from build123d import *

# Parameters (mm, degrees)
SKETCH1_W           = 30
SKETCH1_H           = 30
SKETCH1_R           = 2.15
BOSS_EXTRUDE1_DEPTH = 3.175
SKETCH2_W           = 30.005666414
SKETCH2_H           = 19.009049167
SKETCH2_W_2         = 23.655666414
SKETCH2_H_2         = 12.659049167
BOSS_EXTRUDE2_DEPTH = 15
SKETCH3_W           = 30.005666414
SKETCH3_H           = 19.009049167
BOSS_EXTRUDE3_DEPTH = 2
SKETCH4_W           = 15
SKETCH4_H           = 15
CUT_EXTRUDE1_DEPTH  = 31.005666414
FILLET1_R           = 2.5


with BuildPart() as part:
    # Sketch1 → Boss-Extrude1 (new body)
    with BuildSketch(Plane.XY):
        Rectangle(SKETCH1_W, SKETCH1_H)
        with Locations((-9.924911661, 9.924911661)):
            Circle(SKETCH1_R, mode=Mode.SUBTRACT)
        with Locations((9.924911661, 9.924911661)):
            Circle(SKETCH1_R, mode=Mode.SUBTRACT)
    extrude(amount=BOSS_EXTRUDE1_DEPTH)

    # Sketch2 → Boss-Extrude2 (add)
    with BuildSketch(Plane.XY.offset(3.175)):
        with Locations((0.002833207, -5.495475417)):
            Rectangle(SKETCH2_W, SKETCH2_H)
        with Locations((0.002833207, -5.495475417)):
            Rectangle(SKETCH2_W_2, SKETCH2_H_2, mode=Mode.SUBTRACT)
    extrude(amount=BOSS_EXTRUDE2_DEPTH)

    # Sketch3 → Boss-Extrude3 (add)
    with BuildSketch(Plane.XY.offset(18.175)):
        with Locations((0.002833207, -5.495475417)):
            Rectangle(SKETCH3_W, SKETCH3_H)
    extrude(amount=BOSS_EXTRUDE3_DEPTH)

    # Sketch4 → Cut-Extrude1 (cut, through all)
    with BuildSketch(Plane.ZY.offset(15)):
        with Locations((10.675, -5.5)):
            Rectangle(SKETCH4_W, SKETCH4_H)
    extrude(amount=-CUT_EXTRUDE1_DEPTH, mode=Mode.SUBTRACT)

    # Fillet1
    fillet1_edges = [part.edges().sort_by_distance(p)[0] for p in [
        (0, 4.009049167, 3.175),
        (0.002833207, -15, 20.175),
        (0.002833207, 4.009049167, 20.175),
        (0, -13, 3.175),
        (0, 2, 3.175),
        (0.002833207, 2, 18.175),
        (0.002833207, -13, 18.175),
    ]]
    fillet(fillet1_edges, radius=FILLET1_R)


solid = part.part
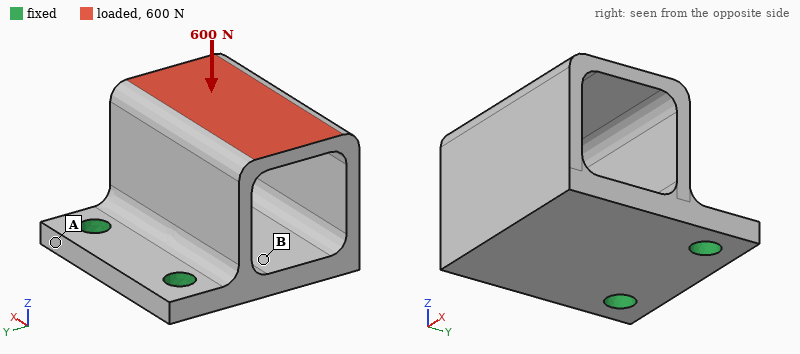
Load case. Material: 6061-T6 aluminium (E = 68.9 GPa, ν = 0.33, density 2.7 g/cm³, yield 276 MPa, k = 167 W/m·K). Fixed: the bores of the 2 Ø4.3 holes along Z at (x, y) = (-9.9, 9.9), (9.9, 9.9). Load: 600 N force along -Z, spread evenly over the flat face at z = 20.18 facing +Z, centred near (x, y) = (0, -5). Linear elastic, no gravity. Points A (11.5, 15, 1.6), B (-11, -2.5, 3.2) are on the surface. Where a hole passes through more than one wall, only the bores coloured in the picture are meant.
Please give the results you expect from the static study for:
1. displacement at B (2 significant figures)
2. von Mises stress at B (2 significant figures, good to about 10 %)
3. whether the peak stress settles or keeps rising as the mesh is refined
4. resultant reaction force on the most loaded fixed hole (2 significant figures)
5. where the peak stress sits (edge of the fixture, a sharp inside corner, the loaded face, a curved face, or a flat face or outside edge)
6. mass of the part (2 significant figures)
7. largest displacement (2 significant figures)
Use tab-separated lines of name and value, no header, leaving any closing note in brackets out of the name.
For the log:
displacement at B	0.070 mm
von Mises stress at B	52 MPa
whether the peak stress settles or keeps rising as the mesh is refined	keeps rising
resultant reaction force on the most loaded fixed hole	300 N
where the peak stress sits	edge of the fixture
mass of the part	16 g
largest displacement	0.26 mm
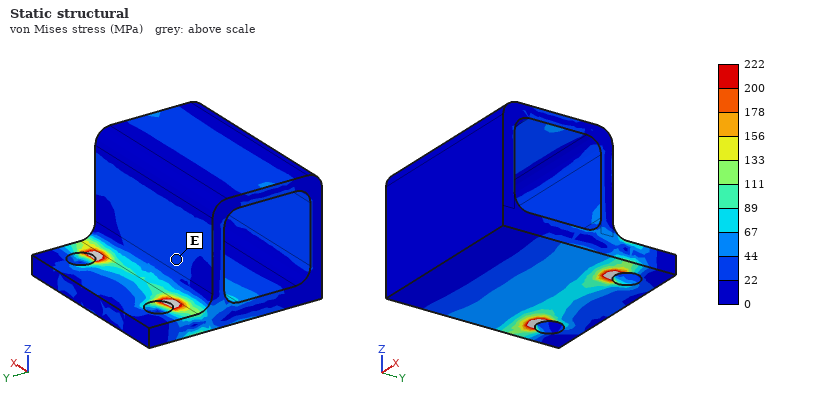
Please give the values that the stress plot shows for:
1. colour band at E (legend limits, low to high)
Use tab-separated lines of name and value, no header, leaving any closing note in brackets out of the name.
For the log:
colour band at E	22 to 44 MPa
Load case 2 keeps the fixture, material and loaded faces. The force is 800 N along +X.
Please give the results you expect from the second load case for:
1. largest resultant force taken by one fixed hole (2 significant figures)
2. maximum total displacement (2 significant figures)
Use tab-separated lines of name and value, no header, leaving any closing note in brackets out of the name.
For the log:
largest resultant force taken by one fixed hole	960 N
maximum total displacement	100 µm
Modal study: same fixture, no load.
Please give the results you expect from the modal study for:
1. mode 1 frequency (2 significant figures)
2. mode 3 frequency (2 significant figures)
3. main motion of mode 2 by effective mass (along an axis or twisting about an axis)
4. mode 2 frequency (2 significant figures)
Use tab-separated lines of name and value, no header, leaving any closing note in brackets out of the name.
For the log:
mode 1 frequency	2200 Hz
mode 3 frequency	8300 Hz
main motion of mode 2 by effective mass	along X
mode 2 frequency	6600 Hz
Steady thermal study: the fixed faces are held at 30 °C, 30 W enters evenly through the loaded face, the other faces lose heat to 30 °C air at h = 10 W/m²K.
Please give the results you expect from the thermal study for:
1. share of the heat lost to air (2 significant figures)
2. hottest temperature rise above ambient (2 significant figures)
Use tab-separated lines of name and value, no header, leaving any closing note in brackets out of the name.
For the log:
share of the heat lost to air	3.5 %
hottest temperature rise above ambient	45 K
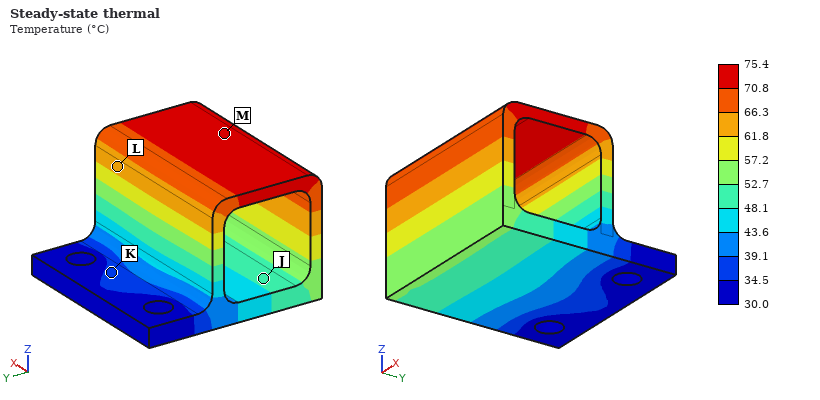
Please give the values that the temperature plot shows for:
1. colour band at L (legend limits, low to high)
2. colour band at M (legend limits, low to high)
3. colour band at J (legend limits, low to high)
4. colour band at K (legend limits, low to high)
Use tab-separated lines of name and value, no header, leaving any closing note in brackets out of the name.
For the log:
colour band at L	61.8 to 66.3 °C
colour band at M	70.8 to 75.4 °C
colour band at J	48.1 to 52.7 °C
colour band at K	34.5 to 39.1 °C
